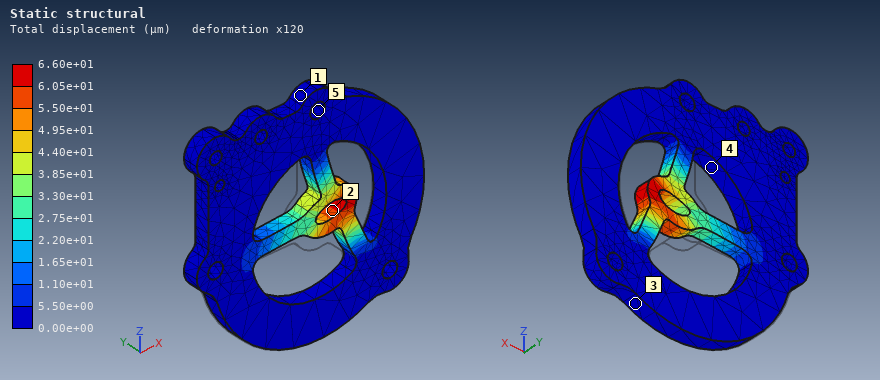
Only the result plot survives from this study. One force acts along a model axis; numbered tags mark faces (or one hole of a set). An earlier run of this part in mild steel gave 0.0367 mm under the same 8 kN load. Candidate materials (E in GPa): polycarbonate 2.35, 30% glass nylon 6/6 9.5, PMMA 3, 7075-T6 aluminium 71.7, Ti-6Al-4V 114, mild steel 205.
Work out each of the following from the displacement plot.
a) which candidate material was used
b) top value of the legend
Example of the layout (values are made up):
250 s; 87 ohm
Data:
Ti-6Al-4V; 6.60e+01 µm
